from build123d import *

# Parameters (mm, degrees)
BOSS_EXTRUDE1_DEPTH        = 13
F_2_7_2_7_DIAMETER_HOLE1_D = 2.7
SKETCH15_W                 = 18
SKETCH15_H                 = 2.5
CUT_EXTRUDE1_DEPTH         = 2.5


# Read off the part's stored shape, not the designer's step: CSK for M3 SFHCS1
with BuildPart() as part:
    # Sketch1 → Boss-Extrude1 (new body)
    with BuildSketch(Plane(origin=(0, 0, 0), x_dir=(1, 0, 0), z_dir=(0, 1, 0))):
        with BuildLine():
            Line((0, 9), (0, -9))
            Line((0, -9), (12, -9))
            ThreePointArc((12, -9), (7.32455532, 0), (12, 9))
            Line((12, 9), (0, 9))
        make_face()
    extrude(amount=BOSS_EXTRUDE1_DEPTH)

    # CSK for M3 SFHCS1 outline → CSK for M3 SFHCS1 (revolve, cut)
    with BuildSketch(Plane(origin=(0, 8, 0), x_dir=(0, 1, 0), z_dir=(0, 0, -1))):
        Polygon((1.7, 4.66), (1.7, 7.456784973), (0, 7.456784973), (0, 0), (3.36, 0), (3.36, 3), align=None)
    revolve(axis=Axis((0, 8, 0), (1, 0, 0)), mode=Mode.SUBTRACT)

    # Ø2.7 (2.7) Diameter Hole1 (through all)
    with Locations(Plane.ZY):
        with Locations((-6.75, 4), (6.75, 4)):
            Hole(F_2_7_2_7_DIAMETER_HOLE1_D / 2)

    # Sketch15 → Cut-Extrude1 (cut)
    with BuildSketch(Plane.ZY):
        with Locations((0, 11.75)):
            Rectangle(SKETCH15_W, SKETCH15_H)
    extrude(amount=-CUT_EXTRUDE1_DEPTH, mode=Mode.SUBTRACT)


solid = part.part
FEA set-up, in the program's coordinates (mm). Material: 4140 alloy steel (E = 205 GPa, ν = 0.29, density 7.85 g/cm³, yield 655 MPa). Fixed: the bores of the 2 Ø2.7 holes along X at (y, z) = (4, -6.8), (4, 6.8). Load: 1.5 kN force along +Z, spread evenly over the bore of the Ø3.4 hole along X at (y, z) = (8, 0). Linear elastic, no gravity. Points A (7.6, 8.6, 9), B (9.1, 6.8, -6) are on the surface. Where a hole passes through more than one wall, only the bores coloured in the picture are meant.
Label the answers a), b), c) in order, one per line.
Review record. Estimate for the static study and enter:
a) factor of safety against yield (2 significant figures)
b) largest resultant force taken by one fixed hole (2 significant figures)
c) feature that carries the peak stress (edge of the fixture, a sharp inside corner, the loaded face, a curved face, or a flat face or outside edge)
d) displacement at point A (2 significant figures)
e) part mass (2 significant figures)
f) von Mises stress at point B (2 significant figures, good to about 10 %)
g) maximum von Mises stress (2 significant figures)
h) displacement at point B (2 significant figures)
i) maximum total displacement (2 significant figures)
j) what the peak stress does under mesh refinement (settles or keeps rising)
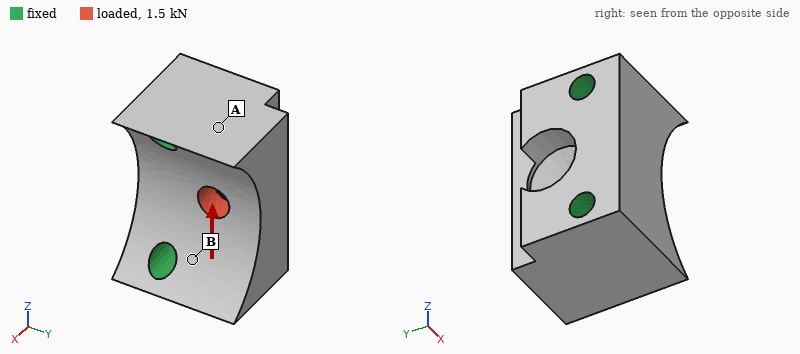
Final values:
a) 7.1
b) 820 N
c) the loaded face
d) 0.80 µm
e) 13 g
f) 21 MPa
g) 92 MPa
h) 0.41 µm
i) 1.8 µm
j) settles
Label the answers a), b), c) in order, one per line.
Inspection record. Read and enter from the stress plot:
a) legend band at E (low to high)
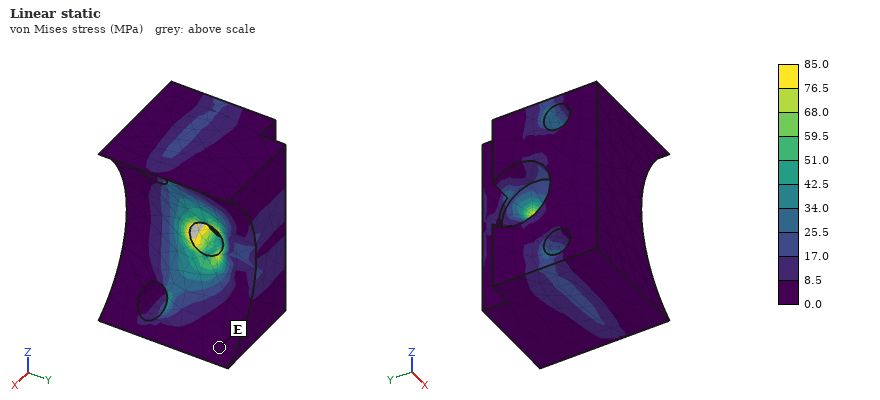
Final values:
a) 0.0 to 8.5 MPa
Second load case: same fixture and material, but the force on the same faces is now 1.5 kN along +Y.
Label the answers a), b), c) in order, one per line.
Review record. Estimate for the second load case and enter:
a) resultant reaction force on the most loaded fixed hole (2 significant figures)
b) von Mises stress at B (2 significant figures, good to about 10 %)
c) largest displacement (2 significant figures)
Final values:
a) 780 N
b) 20 MPa
c) 2.0 µm
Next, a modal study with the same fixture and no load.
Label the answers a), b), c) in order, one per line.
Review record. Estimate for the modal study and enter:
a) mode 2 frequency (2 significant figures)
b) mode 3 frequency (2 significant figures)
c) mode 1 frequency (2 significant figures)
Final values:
a) 66 kHz
b) 78 kHz
c) 65 kHz
